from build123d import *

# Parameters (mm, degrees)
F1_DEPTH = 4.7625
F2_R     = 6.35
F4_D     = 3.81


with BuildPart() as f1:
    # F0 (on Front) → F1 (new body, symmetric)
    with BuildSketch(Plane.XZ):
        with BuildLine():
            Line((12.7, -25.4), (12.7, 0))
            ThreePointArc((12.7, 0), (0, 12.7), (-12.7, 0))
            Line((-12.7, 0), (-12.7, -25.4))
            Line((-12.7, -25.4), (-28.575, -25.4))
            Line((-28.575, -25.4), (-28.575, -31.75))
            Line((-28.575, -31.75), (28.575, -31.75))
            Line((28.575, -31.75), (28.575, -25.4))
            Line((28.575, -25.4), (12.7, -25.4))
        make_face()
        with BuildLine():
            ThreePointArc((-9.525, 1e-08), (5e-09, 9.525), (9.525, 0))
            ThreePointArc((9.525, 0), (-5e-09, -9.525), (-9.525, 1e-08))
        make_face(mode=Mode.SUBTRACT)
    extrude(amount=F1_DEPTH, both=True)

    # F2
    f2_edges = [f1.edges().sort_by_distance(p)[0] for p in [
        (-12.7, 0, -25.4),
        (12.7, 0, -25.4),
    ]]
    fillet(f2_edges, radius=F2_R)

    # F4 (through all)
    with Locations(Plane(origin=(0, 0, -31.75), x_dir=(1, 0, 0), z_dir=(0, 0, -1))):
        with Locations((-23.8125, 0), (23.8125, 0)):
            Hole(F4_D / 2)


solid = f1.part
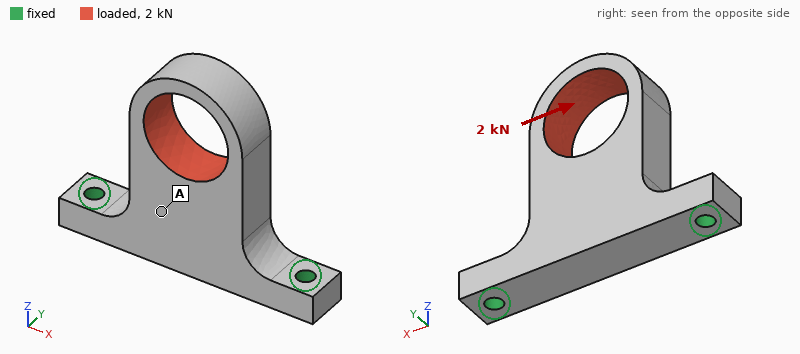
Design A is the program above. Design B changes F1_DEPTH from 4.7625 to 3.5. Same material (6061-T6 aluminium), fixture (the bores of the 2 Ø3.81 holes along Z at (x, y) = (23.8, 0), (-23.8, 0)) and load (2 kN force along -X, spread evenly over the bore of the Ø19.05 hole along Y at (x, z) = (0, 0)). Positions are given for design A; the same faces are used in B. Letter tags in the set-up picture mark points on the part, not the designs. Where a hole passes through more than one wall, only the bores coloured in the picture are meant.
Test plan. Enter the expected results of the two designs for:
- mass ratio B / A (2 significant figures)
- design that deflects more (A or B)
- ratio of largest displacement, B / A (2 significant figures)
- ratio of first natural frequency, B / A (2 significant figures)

0.73
B
1.3
0.86
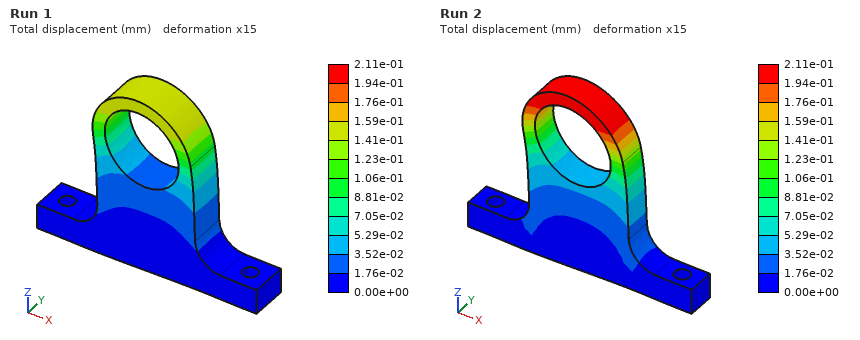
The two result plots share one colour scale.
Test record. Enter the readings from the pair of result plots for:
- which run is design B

Run 2
